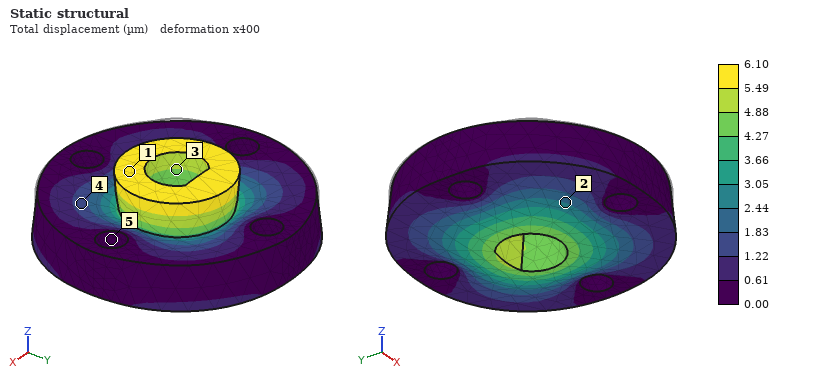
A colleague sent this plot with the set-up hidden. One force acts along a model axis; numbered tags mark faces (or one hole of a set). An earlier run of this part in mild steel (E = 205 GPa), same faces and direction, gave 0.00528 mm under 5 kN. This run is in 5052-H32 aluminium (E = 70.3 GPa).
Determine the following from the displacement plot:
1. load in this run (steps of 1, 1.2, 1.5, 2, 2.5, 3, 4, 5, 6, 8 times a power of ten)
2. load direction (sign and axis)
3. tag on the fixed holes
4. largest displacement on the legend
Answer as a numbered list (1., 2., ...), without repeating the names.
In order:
1. 2 kN
2. -Z
3. 5
4. 6.10 µm
